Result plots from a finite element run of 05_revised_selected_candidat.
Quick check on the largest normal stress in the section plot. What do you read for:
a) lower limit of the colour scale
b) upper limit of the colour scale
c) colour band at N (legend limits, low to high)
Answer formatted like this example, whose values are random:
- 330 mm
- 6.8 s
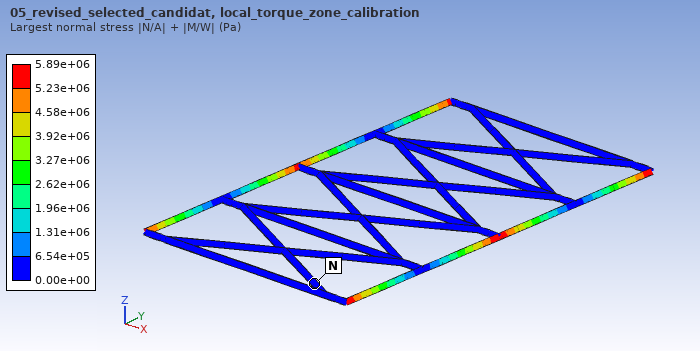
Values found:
- 0.00e+00 Pa
- 5.89e+06 Pa
- 0.00e+00 to 6.54e+05 Pa
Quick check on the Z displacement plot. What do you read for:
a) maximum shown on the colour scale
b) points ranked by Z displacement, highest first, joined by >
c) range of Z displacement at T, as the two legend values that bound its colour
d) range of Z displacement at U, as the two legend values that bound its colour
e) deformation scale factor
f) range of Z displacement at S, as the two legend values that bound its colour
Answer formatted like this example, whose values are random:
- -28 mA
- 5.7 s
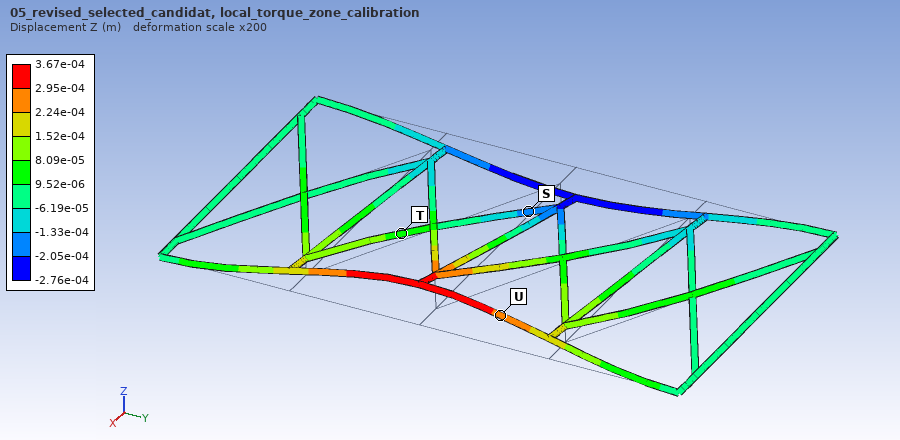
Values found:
- 3.67e-04 m
- U > T > S
- 9.52e-06 to 8.09e-05 m
- 2.24e-04 to 2.95e-04 m
- 200
- -2.05e-04 to -1.33e-04 m
